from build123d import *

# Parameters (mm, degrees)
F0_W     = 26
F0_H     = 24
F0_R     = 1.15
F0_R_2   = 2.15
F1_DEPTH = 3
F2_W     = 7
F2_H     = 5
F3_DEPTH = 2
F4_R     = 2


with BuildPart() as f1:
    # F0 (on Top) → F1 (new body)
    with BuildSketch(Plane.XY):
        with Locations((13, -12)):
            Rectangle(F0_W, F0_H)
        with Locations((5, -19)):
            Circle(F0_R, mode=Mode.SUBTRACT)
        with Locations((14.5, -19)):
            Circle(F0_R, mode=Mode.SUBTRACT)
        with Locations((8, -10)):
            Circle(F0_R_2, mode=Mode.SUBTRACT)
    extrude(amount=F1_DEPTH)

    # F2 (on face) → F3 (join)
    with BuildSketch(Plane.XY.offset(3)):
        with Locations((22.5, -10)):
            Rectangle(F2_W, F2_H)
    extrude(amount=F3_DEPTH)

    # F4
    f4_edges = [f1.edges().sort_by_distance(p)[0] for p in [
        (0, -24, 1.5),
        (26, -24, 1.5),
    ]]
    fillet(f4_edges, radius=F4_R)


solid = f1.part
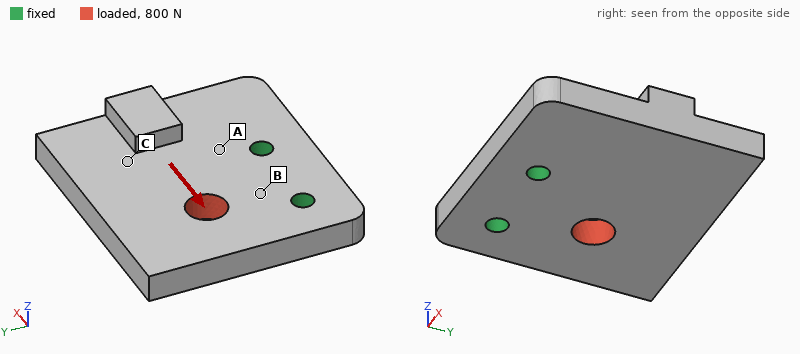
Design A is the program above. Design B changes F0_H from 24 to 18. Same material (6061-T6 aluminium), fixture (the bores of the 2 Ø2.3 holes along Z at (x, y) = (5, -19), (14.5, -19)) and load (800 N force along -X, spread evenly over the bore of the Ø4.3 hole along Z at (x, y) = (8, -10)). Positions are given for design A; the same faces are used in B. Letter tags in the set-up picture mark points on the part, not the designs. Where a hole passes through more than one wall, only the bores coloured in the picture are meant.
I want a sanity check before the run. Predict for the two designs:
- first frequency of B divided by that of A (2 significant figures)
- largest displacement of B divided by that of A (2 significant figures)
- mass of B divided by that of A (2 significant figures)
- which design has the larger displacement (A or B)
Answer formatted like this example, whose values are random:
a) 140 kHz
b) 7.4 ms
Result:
a) 1.3
b) 1.1
c) 0.75
d) B
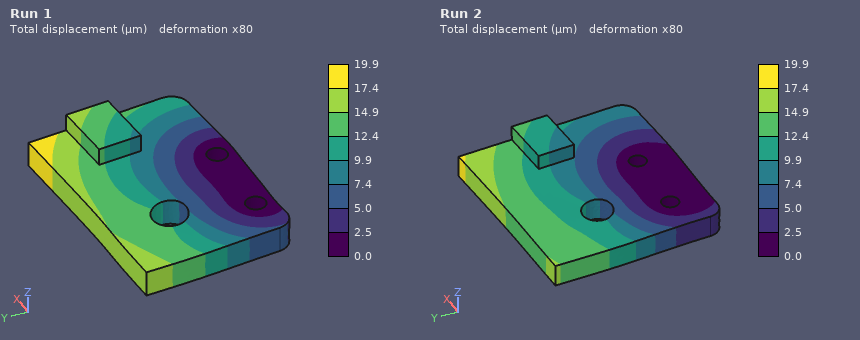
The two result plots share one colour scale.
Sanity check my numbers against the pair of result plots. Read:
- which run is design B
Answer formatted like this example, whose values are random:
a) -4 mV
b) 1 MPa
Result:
a) Run 1
